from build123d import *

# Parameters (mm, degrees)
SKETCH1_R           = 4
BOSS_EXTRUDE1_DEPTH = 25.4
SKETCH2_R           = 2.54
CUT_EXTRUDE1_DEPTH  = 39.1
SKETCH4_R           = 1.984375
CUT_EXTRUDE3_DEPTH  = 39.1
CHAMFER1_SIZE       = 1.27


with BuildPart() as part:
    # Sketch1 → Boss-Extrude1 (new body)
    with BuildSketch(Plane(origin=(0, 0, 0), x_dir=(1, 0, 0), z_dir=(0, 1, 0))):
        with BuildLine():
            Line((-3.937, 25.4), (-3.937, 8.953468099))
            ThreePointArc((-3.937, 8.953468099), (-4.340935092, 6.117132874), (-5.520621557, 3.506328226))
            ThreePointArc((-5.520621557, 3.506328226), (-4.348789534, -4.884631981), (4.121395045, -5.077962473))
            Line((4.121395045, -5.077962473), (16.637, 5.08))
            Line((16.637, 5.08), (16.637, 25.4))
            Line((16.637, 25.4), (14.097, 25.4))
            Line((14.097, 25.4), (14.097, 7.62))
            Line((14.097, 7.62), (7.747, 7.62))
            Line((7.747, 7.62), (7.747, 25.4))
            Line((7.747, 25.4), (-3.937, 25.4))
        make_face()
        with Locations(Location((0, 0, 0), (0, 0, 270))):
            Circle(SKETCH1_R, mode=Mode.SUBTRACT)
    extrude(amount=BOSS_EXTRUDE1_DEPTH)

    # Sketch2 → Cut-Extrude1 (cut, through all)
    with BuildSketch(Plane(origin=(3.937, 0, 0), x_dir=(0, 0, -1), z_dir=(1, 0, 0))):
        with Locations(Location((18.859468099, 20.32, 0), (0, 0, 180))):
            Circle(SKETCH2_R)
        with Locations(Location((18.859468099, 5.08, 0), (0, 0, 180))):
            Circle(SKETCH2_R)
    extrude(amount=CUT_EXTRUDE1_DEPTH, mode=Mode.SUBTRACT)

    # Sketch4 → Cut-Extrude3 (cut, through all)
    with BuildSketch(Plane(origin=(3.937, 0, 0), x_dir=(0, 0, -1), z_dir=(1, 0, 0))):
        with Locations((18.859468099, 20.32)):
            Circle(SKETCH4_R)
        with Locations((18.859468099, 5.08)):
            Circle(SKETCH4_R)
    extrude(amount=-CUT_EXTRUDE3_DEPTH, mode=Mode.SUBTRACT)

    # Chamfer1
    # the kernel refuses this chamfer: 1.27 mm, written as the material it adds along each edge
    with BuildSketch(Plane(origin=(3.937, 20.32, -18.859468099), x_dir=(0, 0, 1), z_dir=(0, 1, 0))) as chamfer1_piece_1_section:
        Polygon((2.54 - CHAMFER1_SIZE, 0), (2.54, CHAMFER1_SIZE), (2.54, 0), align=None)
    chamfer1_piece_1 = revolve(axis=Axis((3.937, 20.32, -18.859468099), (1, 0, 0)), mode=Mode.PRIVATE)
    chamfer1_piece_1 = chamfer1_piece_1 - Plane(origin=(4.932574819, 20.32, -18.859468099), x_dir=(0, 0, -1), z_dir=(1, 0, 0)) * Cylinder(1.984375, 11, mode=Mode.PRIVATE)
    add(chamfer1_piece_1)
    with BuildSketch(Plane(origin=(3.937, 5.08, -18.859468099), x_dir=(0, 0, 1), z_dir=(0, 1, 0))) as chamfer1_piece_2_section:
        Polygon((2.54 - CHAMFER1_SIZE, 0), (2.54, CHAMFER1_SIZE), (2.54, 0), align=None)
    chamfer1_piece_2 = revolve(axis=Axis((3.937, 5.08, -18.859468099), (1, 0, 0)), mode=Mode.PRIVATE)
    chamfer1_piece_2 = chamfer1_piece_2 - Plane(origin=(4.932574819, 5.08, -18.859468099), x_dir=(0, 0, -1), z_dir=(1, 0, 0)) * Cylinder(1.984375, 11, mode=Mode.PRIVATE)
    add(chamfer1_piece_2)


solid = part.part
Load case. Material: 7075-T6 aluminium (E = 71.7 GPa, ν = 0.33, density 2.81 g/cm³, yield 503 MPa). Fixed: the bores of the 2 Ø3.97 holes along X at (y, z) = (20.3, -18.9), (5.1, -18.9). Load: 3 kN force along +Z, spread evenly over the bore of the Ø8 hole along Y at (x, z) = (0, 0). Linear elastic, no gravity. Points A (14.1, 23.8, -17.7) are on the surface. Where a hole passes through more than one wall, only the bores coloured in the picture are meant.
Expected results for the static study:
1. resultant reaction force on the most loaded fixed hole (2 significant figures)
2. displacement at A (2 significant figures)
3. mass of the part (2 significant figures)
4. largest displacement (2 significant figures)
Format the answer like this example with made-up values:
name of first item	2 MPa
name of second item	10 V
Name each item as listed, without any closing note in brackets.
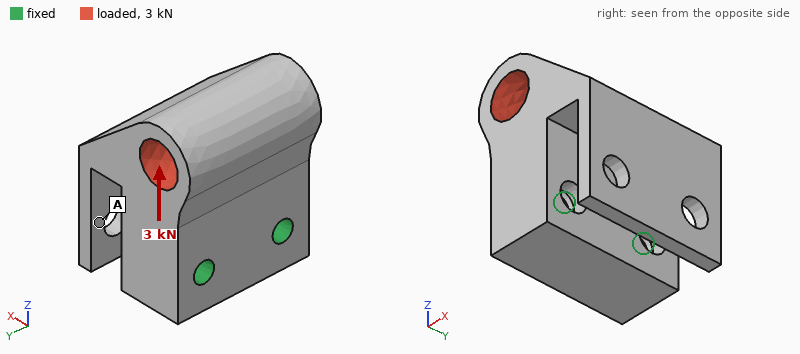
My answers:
resultant reaction force on the most loaded fixed hole	1.5 kN
displacement at A	2.7 µm
mass of the part	29 g
largest displacement	11 µm
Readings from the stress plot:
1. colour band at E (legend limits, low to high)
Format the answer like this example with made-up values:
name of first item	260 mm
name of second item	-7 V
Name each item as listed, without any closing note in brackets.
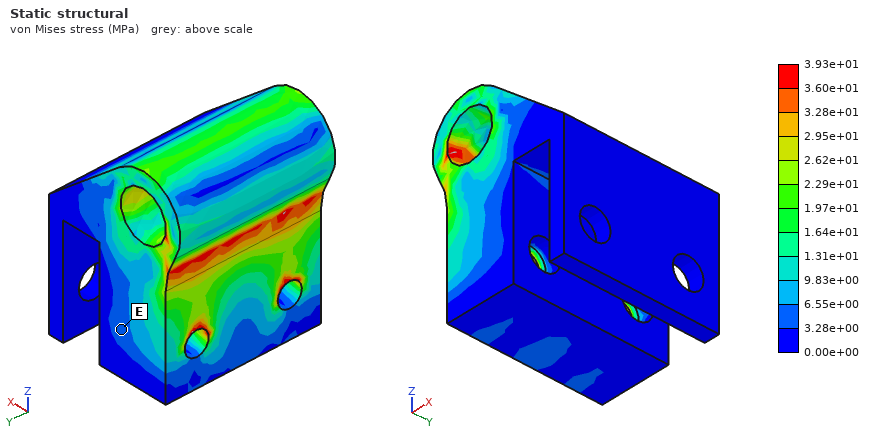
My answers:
colour band at E	3.28e+00 to 6.55e+00 MPa
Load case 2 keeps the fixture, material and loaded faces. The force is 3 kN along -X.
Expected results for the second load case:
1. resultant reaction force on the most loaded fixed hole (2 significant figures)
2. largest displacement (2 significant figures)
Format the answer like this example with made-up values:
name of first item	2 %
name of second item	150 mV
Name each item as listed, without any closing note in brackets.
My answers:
resultant reaction force on the most loaded fixed hole	1.5 kN
largest displacement	77 µm
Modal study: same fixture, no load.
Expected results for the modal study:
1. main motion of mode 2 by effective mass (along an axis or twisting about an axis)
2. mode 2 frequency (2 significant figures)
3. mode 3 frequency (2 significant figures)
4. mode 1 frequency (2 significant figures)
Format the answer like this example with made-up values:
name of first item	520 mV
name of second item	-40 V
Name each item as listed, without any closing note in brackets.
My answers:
main motion of mode 2 by effective mass	along X
mode 2 frequency	9700 Hz
mode 3 frequency	10 kHz
mode 1 frequency	5500 Hz
